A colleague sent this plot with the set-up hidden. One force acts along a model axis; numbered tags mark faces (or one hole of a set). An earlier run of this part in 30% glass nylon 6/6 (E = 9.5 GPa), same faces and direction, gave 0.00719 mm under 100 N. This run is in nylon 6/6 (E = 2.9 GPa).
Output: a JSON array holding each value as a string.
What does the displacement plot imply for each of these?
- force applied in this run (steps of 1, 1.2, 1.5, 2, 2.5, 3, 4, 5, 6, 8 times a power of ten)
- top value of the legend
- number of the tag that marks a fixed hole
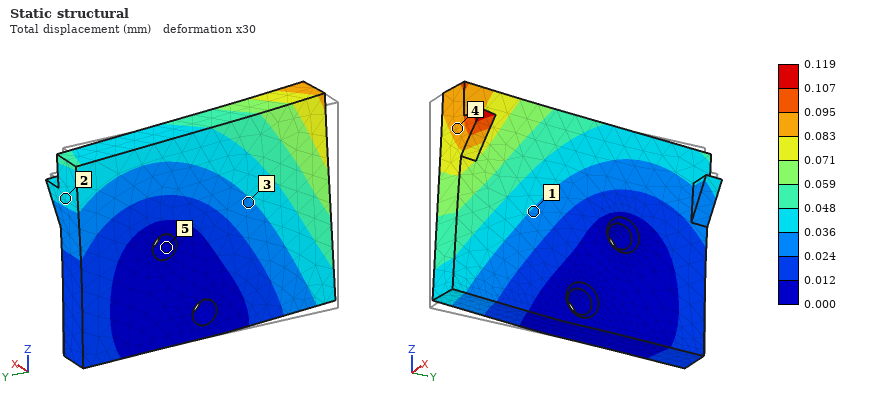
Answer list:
["500 N", "0.119 mm", "5"]
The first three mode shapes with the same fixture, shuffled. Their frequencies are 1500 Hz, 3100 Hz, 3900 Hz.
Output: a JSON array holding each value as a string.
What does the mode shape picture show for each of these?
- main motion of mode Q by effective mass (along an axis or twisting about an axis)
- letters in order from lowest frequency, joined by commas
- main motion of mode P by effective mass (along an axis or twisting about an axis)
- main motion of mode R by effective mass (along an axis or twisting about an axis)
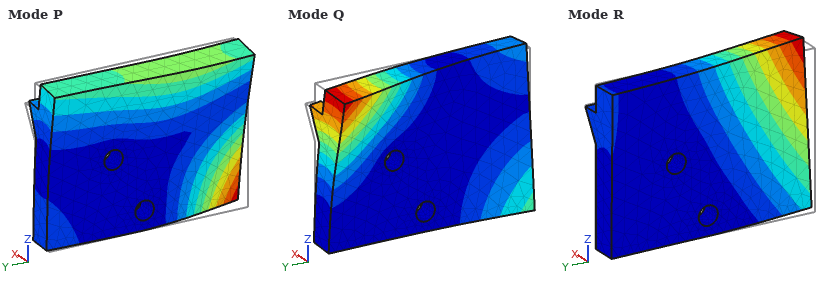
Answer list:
["along X", "R, P, Q", "twisting about Y", "along X"]
